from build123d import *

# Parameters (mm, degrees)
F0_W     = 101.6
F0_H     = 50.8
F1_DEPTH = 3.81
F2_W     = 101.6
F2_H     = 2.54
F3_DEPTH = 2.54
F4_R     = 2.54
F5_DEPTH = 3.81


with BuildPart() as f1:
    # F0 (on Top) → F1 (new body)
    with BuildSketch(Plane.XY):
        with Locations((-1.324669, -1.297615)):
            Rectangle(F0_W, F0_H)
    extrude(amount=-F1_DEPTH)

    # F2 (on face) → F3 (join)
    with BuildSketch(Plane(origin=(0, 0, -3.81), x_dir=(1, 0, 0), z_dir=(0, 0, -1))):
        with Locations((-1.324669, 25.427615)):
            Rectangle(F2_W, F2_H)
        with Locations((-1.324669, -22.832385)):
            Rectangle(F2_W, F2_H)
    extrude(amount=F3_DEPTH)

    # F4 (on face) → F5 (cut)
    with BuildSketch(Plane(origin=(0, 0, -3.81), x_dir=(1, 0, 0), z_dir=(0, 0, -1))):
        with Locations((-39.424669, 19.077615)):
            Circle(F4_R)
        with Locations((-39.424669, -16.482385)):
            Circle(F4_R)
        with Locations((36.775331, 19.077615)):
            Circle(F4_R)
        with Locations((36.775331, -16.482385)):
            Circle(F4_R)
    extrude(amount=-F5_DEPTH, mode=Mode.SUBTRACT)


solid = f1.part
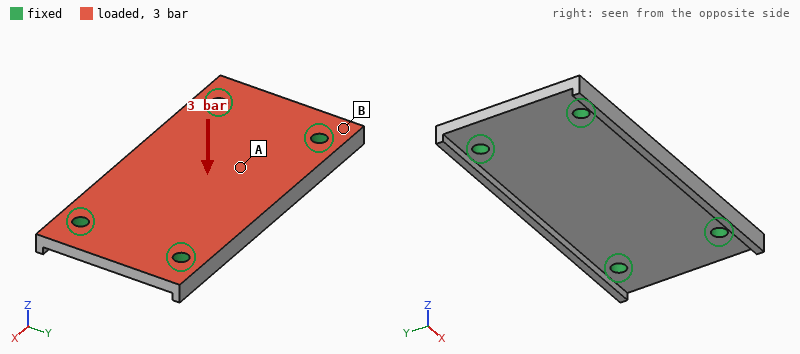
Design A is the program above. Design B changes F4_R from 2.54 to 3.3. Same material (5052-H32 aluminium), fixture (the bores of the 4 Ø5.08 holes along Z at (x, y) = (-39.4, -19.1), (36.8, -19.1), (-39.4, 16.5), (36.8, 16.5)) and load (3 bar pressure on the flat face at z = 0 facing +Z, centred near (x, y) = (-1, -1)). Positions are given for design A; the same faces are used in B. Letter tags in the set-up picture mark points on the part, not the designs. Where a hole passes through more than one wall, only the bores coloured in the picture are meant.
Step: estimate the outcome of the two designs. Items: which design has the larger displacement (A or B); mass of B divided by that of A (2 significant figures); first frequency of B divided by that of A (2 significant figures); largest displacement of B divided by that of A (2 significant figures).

A
0.99
1.1
0.90
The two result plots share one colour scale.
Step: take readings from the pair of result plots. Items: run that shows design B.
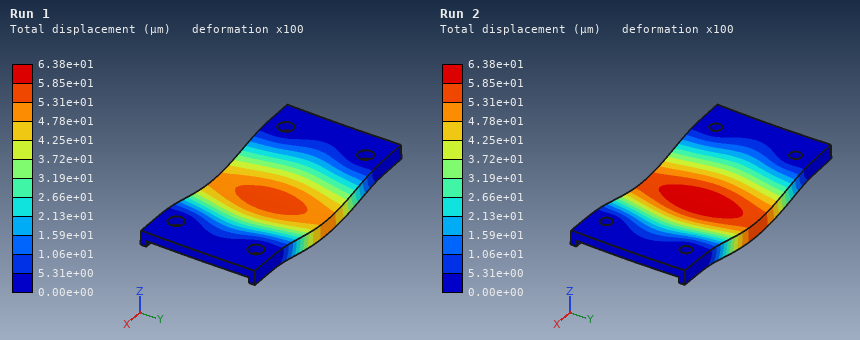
Run 1
